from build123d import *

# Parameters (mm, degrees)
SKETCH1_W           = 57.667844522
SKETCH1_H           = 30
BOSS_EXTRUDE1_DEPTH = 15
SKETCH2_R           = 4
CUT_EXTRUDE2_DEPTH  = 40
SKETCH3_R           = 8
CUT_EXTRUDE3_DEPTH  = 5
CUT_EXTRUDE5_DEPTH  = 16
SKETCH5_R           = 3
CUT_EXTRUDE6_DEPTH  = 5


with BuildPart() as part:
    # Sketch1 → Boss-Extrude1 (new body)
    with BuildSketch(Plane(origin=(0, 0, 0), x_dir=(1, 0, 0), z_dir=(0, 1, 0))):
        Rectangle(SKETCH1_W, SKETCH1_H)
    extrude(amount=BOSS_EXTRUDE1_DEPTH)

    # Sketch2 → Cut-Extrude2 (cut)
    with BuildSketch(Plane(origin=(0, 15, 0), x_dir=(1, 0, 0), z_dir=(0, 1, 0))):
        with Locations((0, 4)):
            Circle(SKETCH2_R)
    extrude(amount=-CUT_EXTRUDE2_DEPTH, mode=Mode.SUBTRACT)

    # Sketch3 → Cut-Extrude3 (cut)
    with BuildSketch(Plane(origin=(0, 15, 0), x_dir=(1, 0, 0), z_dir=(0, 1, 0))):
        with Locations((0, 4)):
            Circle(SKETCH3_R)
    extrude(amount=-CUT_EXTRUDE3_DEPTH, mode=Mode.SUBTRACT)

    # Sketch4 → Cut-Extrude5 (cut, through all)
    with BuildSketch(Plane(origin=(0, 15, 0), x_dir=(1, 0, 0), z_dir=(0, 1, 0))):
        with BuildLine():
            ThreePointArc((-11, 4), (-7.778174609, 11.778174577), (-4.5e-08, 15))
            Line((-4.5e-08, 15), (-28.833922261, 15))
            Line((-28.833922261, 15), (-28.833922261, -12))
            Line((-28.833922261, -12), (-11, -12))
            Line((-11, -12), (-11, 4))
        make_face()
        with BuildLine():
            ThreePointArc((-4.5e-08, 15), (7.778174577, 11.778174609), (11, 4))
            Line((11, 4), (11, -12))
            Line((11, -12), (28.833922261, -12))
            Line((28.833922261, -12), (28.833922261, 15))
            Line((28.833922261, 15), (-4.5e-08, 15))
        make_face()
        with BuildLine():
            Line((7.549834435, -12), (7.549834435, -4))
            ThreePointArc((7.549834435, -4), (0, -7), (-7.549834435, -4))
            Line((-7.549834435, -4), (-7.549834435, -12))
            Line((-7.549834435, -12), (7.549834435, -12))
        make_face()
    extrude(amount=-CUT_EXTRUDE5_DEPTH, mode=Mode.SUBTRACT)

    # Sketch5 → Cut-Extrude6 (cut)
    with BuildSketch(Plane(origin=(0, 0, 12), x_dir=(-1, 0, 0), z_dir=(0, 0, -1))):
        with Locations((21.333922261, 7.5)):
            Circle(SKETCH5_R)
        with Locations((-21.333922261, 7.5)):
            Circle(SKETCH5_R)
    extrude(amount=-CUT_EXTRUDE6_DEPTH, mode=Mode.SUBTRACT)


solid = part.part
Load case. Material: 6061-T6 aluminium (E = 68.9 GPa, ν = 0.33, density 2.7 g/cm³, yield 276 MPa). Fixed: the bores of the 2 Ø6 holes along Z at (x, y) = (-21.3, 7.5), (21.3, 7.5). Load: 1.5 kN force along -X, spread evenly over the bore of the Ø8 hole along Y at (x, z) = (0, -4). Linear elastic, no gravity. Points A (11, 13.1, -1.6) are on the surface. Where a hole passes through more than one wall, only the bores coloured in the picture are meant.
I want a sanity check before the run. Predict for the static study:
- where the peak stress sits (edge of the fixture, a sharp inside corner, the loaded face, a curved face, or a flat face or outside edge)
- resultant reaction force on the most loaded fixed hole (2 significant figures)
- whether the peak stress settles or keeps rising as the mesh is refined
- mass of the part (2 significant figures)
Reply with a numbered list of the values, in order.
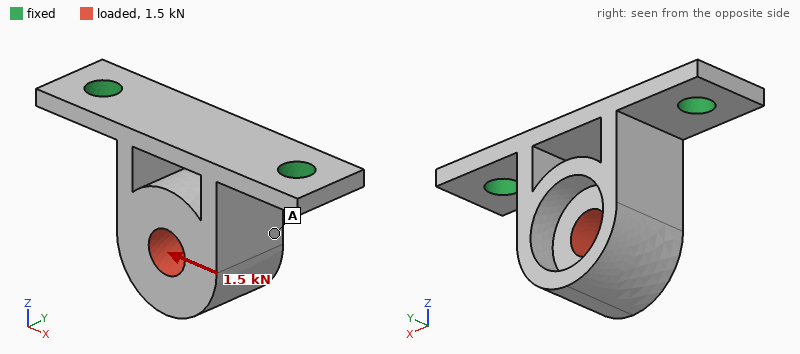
1. edge of the fixture
2. 1.1 kN
3. keeps rising
4. 21 g
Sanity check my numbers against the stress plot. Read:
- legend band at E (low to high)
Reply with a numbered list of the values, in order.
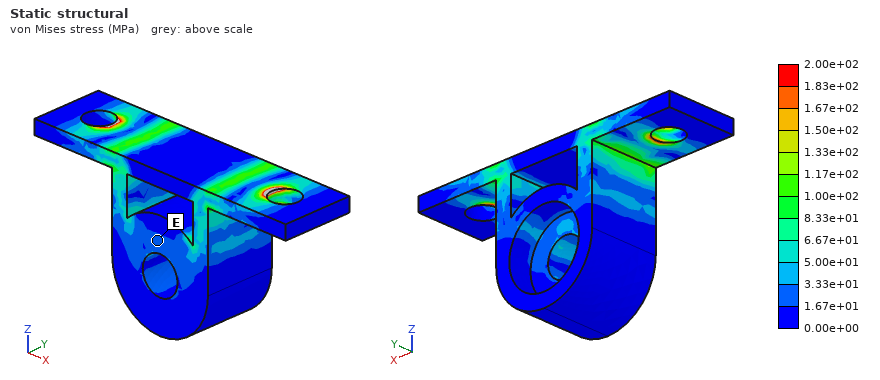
1. 1.67e+01 to 3.33e+01 MPa
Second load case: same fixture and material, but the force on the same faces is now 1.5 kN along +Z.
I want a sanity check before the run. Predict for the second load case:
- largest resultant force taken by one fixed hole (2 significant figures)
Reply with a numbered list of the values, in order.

1. 790 N
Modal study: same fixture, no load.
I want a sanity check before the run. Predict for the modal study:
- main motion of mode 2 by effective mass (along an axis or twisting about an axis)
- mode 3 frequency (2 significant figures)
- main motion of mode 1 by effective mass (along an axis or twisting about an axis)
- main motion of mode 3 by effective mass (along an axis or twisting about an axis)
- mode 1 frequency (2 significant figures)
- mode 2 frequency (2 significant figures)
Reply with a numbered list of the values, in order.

1. along X
2. 7200 Hz
3. along Y
4. along Z
5. 2300 Hz
6. 6200 Hz
